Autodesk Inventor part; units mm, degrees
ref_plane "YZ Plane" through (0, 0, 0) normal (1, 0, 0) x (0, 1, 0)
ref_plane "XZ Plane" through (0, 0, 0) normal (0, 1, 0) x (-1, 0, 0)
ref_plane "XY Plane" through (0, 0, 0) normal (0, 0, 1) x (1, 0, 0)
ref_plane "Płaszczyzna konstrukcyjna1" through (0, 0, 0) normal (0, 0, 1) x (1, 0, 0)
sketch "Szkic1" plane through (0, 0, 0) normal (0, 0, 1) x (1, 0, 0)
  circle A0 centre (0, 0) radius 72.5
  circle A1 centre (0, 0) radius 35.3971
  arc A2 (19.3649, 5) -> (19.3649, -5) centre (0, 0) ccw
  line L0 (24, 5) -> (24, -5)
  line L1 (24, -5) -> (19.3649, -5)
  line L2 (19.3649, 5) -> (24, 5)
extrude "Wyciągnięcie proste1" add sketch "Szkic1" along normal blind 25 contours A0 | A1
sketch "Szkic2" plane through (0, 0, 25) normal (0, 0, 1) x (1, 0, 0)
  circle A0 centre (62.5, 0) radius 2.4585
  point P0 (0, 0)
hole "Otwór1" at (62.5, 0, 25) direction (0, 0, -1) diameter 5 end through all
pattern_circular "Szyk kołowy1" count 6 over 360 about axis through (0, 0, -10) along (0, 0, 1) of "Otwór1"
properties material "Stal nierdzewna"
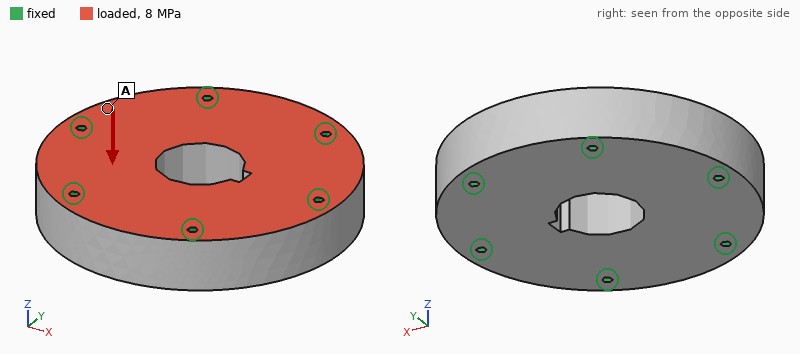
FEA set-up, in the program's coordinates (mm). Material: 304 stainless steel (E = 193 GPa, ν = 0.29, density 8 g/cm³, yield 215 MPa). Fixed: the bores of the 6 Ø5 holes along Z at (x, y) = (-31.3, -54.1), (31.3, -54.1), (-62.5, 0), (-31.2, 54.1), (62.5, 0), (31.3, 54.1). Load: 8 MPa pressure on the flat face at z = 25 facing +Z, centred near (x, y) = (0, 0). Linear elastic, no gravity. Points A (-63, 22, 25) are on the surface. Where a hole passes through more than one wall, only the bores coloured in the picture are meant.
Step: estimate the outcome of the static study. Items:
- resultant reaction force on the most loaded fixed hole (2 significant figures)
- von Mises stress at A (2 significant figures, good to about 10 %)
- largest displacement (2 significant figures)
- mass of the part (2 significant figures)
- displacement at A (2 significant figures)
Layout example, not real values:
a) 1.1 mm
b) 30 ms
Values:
a) 20 kN
b) 18 MPa
c) 18 µm
d) 3.0 kg
e) 5.1 µm
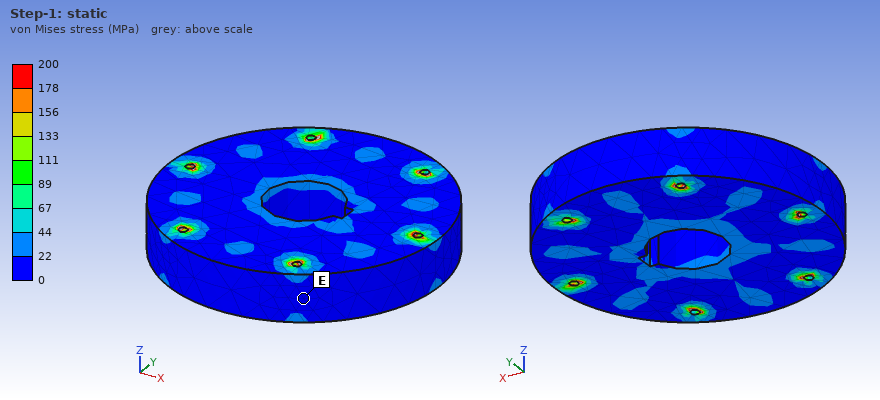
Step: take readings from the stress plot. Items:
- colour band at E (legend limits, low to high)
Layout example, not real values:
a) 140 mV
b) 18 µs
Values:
a) 0 to 22 MPa
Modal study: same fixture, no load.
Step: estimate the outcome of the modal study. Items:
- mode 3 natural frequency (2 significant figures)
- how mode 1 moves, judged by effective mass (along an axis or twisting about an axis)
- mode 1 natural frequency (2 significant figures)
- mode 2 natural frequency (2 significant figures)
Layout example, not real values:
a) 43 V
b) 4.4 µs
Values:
a) 14 kHz
b) along Z
c) 9100 Hz
d) 14 kHz
